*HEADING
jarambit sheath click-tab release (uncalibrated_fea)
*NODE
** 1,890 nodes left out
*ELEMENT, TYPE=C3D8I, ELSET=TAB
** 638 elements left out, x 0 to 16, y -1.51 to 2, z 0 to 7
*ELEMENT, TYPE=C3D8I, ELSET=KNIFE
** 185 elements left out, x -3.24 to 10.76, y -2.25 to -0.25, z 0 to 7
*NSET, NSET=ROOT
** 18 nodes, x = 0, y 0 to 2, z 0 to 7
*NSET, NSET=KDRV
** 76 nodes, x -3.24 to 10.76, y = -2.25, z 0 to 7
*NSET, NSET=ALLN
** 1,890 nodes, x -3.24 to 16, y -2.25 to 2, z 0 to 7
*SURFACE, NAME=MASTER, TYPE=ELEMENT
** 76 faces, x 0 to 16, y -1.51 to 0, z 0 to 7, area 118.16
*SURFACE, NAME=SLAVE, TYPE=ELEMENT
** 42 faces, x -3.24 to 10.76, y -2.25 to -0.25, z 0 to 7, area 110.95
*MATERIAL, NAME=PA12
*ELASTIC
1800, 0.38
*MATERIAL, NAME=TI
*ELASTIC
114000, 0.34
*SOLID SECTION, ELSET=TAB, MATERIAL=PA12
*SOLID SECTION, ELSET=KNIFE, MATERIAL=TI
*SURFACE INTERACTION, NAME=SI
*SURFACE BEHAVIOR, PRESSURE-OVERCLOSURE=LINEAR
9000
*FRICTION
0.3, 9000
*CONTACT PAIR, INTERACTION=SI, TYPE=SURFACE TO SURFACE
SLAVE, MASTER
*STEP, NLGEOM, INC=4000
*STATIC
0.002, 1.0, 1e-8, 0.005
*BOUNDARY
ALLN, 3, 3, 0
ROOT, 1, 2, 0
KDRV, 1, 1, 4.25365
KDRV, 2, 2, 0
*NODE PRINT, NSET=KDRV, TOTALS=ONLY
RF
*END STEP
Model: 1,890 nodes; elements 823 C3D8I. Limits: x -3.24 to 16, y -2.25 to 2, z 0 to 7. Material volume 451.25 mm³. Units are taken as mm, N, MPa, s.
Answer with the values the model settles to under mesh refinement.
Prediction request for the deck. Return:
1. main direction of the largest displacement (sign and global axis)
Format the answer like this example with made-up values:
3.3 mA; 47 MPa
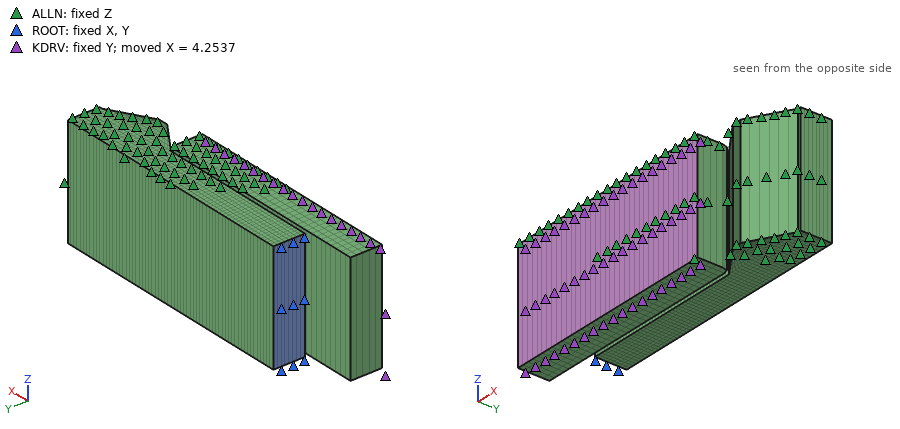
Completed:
+X
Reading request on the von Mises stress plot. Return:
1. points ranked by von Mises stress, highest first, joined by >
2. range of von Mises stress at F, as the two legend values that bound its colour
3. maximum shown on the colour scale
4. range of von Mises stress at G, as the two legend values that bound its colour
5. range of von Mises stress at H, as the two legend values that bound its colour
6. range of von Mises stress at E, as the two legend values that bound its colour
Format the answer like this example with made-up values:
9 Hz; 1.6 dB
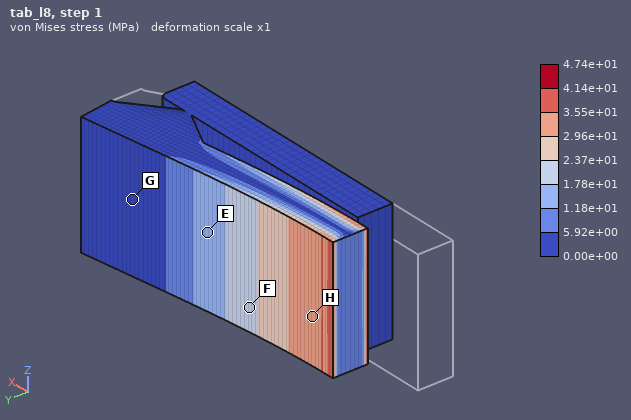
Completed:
H > F > E > G; 1.78e+01 to 2.37e+01 MPa; 4.74e+01 MPa; 0.00e+00 to 5.92e+00 MPa; 2.96e+01 to 3.55e+01 MPa; 1.18e+01 to 1.78e+01 MPa
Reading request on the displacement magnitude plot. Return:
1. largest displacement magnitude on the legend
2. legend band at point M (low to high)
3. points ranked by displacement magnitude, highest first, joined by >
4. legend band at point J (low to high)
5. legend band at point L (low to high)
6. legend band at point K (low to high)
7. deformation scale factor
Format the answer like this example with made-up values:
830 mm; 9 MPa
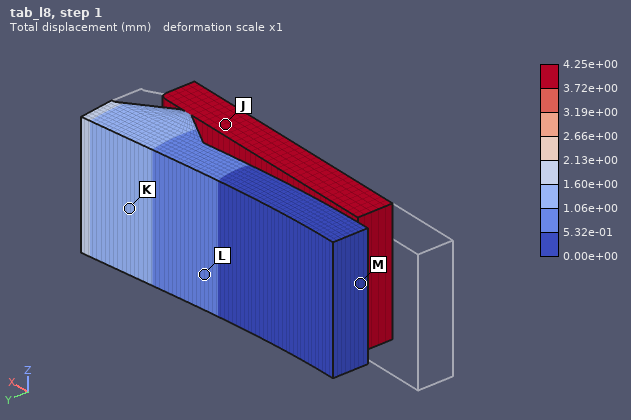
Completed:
4.25e+00 mm; 0.00e+00 to 5.32e-01 mm; J > K > L > M; 3.72e+00 to 4.25e+00 mm; 5.32e-01 to 1.06e+00 mm; 1.06e+00 to 1.60e+00 mm; 1
